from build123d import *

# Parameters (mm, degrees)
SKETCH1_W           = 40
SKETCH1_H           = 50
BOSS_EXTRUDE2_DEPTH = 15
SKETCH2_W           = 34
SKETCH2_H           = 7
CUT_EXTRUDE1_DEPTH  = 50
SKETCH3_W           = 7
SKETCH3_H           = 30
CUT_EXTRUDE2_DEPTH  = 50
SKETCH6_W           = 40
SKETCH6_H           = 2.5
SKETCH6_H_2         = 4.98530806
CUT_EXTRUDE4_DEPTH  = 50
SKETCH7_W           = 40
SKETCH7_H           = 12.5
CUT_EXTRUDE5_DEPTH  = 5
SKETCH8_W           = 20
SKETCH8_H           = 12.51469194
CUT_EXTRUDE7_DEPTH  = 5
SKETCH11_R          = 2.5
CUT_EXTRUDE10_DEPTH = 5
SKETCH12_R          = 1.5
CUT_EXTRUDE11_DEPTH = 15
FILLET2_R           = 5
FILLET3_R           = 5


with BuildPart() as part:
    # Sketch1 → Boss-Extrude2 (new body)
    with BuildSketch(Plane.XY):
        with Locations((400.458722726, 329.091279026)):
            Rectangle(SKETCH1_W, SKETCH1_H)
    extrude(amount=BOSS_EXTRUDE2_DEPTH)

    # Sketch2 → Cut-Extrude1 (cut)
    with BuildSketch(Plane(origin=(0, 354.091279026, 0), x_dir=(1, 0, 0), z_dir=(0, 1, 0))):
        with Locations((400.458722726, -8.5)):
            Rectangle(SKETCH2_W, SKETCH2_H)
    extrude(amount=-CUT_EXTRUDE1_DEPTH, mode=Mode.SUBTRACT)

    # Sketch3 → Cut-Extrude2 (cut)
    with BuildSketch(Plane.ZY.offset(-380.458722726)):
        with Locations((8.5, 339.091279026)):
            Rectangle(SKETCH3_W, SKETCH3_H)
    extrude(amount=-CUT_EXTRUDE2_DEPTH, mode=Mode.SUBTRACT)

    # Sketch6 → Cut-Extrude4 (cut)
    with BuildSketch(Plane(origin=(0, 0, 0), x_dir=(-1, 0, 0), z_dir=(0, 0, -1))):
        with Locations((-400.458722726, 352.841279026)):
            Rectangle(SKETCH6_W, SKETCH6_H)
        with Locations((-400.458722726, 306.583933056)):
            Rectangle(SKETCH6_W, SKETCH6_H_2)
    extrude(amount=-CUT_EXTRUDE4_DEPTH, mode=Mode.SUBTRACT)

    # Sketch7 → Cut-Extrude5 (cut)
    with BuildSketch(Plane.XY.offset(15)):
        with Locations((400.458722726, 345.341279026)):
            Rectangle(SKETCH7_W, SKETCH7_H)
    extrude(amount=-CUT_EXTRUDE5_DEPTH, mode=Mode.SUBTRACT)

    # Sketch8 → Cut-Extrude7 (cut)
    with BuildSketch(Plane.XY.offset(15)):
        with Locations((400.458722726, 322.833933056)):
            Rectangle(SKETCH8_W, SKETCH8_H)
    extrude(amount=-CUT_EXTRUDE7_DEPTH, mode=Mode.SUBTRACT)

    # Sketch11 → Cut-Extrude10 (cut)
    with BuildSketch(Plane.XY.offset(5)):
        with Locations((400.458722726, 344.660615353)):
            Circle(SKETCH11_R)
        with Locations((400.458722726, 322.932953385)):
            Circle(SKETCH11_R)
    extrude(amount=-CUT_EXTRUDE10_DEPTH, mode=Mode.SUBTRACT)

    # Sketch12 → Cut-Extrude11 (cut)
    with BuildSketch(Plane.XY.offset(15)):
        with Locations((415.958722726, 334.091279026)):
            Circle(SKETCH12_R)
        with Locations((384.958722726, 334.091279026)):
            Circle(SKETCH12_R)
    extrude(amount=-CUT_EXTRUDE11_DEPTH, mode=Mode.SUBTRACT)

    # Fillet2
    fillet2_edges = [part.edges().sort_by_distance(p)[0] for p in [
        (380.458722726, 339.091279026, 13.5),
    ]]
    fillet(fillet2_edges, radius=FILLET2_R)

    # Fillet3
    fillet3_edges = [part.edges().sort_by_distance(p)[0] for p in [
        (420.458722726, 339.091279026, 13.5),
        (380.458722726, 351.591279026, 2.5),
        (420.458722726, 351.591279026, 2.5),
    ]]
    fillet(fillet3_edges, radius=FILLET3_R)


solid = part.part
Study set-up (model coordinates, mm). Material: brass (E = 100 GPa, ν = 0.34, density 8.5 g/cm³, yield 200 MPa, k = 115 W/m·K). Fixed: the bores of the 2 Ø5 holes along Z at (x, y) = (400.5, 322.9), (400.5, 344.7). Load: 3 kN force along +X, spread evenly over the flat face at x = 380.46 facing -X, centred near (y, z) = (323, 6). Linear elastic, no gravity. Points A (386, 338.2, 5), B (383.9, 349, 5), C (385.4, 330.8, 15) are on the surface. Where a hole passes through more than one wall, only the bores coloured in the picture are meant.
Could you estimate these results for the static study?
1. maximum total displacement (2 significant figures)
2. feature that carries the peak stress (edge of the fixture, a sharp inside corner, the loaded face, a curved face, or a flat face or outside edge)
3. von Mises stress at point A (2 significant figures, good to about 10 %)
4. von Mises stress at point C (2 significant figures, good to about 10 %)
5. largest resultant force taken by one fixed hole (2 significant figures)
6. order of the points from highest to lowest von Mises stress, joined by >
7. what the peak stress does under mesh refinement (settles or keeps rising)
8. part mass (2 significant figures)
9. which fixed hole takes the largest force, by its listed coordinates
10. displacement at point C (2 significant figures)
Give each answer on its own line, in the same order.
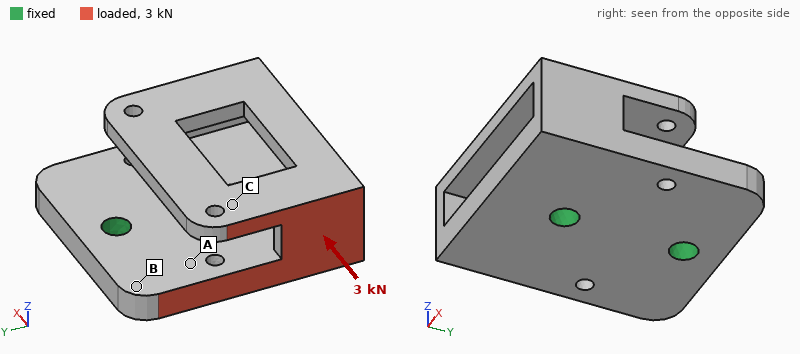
84 µm
edge of the fixture
25 MPa
40 MPa
2.8 kN
C > A > B
keeps rising
99 g
(400.5, 322.9)
73 µm
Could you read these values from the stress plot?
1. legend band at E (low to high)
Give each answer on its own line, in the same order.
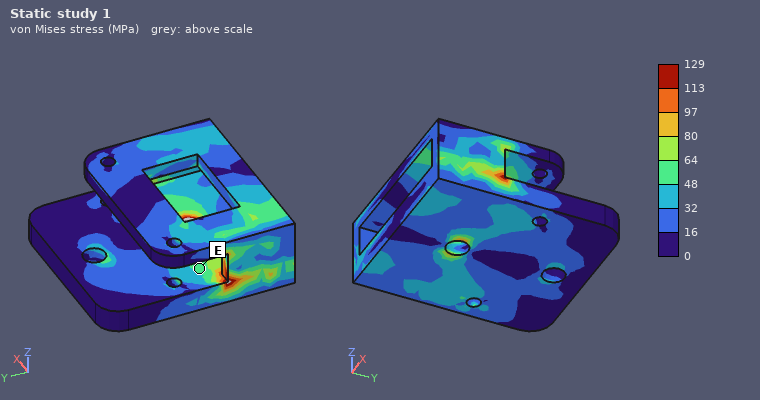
48 to 64 MPa
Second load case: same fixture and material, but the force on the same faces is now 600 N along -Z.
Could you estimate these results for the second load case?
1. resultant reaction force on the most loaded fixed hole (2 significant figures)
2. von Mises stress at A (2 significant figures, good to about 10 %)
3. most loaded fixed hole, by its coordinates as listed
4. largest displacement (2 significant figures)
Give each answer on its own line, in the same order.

520 N
20 MPa
(400.5, 322.9)
48 µm
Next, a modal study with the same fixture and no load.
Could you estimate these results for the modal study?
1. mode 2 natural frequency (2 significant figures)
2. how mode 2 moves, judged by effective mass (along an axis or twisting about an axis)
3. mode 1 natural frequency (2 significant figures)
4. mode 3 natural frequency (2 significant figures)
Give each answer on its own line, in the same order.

3300 Hz
along X
2700 Hz
4200 Hz
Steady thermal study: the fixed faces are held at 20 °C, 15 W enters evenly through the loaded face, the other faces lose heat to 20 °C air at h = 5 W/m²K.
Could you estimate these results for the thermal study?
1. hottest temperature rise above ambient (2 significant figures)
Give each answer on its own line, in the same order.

21 K
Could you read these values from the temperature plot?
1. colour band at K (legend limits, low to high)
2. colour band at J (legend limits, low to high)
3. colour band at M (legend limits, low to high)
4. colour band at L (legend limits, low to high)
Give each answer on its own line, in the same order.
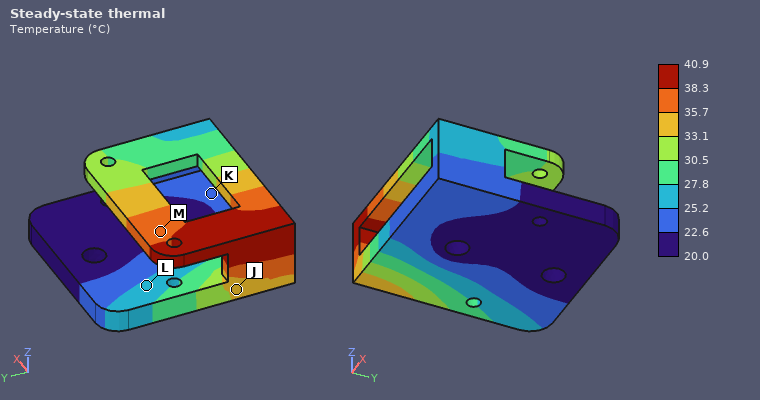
22.6 to 25.2 °C
33.1 to 35.7 °C
35.7 to 38.3 °C
25.2 to 27.8 °C
